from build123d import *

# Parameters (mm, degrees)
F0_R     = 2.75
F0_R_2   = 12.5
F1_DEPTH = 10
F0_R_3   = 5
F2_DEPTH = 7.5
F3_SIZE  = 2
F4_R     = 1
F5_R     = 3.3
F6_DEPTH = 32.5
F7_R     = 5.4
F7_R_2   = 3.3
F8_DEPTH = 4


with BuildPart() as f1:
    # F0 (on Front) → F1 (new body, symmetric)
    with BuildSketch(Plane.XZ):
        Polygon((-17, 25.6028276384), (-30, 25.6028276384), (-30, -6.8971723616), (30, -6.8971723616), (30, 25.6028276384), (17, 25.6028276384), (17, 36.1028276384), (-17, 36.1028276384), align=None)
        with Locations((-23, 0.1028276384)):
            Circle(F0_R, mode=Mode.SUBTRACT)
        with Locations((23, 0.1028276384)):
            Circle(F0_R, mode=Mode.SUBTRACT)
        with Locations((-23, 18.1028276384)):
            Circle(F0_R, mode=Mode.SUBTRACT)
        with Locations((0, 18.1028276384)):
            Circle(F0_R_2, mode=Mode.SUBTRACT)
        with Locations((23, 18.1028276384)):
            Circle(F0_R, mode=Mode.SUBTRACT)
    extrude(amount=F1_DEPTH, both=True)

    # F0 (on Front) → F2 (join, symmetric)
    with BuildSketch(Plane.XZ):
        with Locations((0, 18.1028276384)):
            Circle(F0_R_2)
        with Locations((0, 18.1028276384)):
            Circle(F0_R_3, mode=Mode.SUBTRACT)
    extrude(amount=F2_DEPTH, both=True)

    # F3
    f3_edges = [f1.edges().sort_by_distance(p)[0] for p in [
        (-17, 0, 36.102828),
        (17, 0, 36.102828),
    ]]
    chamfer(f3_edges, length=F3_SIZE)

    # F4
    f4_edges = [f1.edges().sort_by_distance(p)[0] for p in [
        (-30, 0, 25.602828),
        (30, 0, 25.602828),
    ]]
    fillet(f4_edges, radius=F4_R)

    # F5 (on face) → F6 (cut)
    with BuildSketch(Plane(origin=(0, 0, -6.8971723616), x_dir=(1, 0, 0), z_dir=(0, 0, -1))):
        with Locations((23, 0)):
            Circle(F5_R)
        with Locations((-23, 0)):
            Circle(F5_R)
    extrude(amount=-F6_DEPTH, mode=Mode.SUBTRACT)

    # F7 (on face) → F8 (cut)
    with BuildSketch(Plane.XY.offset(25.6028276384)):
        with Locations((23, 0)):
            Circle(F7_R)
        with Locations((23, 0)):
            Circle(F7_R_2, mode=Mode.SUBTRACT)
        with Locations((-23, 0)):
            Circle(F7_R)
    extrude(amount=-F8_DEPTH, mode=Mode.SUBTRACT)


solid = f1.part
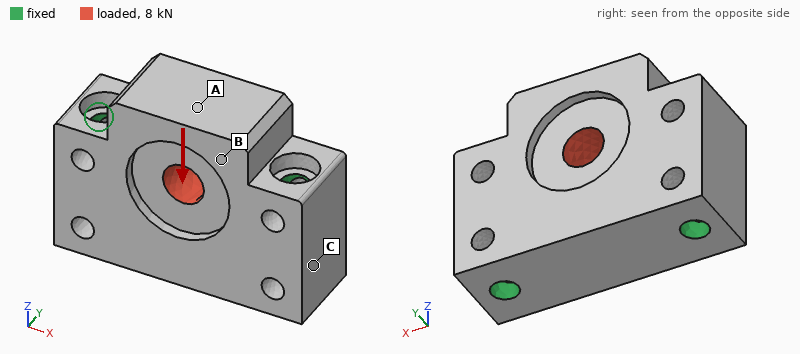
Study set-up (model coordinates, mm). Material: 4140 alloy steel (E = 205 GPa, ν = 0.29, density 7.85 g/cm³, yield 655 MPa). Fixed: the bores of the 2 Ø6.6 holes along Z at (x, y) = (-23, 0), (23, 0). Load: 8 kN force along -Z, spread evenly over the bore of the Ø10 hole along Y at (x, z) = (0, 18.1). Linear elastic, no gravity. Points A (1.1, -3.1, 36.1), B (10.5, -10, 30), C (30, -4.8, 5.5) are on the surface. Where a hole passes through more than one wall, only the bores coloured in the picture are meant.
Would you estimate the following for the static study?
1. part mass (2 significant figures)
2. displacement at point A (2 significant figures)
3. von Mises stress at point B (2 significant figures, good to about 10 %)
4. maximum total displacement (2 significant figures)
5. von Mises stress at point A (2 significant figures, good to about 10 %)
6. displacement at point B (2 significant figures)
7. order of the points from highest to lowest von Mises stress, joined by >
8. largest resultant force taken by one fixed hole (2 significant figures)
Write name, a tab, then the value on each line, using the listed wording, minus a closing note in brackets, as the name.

part mass	300 g
displacement at point A	1.9 µm
von Mises stress at point B	8.3 MPa
maximum total displacement	2.5 µm
von Mises stress at point A	13 MPa
displacement at point B	1.5 µm
order of the points from highest to lowest von Mises stress, joined by >	A > B > C
largest resultant force taken by one fixed hole	4.1 kN
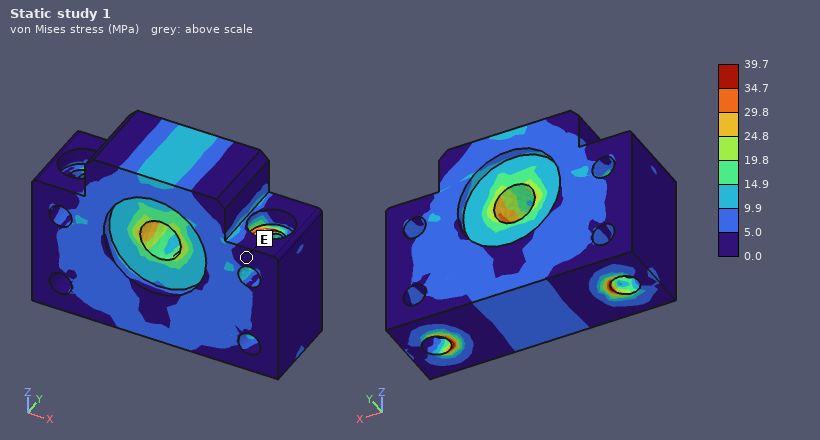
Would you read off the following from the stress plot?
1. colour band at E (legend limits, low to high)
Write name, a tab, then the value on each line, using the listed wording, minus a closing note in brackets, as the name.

colour band at E	0.0 to 5.0 MPa
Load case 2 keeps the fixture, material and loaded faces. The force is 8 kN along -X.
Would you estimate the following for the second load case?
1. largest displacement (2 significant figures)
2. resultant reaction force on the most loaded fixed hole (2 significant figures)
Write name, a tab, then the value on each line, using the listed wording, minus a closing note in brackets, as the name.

largest displacement	1.9 µm
resultant reaction force on the most loaded fixed hole	4.1 kN
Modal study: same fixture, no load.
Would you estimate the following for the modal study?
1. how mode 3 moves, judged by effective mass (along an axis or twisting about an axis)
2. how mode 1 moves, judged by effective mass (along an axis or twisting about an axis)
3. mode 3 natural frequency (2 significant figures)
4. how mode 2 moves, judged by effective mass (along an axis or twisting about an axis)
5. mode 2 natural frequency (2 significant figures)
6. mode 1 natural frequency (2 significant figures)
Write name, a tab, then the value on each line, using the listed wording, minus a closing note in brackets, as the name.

how mode 3 moves, judged by effective mass	along Z
how mode 1 moves, judged by effective mass	along Y
mode 3 natural frequency	28 kHz
how mode 2 moves, judged by effective mass	along Y
mode 2 natural frequency	25 kHz
mode 1 natural frequency	14 kHz
